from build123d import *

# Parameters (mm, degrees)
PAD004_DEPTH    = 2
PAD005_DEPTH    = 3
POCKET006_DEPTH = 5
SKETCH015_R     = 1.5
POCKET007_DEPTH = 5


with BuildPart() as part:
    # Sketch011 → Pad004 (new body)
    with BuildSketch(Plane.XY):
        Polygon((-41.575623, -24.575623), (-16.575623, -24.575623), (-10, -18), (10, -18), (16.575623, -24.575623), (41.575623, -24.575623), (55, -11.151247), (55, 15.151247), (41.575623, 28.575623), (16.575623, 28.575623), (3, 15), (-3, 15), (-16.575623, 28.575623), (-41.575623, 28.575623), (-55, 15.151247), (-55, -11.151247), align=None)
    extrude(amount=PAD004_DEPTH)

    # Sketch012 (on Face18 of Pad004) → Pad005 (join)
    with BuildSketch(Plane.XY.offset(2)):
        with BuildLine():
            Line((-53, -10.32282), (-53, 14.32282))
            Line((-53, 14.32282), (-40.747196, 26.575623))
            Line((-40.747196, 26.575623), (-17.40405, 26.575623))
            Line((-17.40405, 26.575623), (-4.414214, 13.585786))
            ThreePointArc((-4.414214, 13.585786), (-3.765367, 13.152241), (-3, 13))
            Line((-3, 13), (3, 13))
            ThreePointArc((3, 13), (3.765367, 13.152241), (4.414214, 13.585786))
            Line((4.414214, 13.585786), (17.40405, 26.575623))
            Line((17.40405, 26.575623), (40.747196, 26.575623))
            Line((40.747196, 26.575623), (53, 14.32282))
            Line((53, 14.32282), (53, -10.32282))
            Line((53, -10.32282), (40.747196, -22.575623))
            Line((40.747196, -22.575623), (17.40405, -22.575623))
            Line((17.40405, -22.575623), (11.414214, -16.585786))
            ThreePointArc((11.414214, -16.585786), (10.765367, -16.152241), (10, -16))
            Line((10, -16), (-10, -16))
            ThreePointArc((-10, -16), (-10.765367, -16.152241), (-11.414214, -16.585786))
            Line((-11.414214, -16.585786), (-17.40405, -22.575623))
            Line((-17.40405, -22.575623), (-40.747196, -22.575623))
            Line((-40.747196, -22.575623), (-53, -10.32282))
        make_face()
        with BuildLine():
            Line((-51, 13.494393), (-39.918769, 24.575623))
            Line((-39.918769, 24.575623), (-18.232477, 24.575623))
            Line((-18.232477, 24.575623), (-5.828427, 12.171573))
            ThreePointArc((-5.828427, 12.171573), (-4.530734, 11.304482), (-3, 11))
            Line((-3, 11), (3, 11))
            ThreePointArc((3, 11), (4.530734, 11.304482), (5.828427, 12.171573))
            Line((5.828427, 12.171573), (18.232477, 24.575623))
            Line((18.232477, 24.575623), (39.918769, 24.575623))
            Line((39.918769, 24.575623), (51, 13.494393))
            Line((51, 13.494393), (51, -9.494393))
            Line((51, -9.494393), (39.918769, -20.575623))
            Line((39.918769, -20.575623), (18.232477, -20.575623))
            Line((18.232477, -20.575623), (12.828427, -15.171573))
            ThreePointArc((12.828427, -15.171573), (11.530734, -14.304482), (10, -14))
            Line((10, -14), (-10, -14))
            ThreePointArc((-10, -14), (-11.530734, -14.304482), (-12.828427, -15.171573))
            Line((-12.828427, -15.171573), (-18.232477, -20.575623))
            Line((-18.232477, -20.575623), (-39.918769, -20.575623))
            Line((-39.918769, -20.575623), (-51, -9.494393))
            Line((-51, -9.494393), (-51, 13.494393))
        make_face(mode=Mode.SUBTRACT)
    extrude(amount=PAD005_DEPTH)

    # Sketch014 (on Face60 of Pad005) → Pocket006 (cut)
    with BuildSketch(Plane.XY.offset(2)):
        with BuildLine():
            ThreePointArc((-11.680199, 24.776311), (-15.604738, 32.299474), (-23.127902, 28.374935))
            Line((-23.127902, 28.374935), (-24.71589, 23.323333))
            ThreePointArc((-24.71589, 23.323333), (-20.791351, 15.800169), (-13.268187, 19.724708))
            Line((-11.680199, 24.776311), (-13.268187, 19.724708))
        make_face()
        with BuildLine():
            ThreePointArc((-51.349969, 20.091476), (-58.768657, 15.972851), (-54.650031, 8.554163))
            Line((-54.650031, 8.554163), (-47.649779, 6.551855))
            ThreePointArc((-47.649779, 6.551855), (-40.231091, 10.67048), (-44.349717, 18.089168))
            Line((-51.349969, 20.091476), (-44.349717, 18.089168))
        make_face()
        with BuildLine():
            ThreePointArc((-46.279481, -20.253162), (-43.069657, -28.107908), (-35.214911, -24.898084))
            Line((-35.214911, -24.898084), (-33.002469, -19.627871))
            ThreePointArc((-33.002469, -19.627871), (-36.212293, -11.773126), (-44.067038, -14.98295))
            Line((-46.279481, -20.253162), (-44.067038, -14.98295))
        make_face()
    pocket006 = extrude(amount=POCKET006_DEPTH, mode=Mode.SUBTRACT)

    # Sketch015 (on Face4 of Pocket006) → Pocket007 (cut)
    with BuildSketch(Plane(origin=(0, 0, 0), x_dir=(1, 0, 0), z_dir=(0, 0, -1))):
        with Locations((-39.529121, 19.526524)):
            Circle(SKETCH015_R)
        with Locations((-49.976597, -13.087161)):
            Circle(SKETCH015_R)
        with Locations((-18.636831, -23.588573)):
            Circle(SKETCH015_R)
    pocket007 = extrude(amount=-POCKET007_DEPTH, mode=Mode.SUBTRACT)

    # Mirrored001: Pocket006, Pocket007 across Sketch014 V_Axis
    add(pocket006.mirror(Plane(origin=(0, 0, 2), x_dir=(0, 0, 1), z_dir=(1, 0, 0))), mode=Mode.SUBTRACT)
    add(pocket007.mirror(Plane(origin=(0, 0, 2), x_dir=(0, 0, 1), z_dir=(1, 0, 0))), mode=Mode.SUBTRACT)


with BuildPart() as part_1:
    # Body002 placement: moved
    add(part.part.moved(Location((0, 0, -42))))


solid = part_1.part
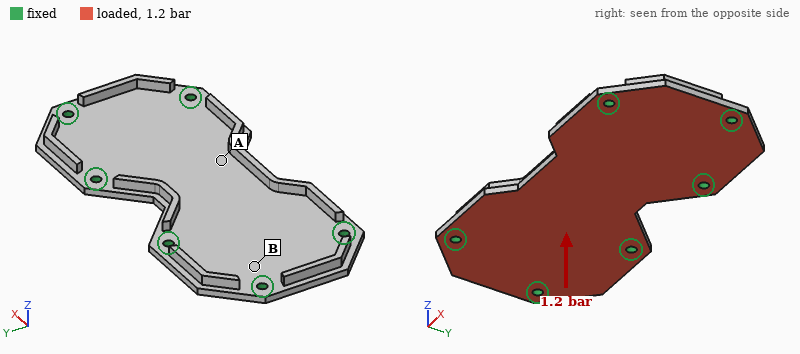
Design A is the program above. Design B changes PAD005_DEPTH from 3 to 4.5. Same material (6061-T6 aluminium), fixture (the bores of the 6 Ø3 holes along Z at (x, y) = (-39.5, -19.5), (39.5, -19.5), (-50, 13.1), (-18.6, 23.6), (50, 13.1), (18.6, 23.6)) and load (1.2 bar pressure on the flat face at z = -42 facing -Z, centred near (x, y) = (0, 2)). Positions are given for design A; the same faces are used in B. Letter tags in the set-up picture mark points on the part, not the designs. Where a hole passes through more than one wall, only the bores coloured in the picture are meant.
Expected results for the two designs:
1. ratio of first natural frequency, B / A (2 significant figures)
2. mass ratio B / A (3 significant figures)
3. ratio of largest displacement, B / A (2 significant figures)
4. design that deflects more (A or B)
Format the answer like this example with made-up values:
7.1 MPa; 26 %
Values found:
1.1; 1.06; 0.81; A
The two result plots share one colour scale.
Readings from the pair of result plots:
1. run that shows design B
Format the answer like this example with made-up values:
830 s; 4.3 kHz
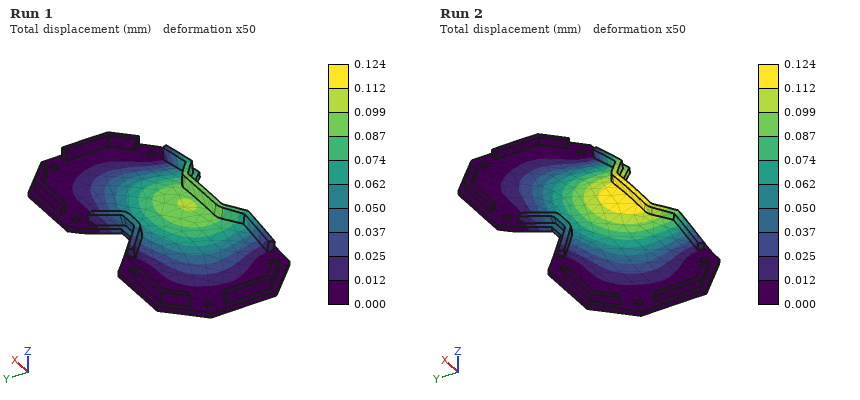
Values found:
Run 1
